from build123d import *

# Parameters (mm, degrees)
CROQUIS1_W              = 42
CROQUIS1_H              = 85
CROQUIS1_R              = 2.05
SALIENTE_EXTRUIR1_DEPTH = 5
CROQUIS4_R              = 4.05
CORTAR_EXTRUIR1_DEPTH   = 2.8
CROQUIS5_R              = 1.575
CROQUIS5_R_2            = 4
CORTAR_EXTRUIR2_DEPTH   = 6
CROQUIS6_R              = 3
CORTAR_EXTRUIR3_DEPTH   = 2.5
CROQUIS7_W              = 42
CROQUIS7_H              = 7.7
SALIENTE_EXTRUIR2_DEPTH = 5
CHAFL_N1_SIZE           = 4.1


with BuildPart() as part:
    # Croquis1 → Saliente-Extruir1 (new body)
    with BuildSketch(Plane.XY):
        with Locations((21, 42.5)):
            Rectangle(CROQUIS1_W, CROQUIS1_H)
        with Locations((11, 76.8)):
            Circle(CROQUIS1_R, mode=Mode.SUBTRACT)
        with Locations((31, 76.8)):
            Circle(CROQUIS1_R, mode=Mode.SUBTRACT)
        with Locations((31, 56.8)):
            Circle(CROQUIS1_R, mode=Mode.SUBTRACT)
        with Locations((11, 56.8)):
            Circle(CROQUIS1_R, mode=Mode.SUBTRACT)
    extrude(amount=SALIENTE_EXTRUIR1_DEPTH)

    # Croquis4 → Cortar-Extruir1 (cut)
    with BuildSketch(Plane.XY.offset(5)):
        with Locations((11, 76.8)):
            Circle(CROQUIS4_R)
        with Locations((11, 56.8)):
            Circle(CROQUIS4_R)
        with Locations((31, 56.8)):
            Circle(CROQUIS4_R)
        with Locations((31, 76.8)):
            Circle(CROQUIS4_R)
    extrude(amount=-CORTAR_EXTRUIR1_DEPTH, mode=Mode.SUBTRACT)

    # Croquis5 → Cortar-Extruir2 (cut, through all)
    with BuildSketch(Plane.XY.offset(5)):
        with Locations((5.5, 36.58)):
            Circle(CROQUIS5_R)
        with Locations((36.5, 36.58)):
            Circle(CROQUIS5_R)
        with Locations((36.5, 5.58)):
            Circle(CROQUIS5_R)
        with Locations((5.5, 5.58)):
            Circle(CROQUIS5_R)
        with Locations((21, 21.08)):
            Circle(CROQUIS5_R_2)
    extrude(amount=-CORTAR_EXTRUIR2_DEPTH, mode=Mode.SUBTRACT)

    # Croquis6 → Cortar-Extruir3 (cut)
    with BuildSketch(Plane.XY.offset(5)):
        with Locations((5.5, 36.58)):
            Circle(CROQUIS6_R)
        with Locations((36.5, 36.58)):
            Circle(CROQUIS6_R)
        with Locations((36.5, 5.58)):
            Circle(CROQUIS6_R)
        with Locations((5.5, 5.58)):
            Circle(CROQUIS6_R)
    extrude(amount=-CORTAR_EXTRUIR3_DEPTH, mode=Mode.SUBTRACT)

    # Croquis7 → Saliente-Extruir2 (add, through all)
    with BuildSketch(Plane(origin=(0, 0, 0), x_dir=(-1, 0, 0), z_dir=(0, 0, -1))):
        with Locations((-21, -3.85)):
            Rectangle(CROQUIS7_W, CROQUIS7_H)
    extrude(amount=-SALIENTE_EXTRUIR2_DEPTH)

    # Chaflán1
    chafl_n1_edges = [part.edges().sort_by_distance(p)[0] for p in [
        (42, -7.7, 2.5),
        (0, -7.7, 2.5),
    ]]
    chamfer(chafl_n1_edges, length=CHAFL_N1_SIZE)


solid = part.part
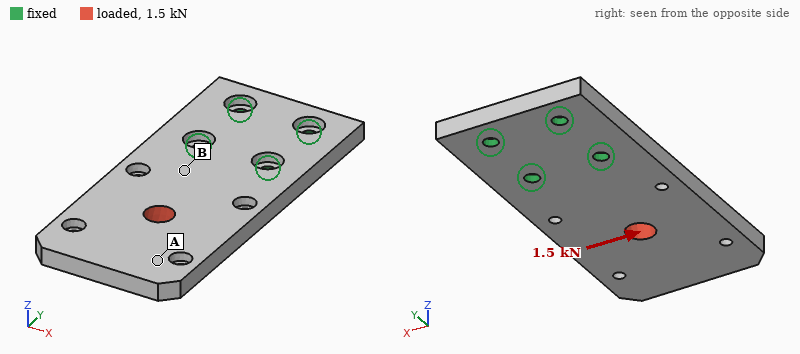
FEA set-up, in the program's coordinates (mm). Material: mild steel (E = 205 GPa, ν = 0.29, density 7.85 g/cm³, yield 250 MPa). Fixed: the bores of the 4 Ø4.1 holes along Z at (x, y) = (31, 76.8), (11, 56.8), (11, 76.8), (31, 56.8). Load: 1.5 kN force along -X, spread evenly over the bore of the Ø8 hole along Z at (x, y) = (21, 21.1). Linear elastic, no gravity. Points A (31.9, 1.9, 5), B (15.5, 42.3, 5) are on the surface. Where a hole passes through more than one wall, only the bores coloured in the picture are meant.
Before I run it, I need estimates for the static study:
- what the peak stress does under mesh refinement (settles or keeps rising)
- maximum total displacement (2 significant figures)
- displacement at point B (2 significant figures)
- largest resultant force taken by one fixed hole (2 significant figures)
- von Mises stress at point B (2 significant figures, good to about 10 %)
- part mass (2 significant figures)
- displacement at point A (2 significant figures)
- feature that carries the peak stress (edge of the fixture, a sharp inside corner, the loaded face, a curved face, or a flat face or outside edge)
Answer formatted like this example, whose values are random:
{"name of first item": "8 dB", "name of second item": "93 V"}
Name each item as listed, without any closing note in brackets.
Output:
{"what the peak stress does under mesh refinement": "keeps rising", "maximum total displacement": "20 µm", "displacement at point B": "4.1 µm", "largest resultant force taken by one fixed hole": "1.7 kN", "von Mises stress at point B": "18 MPa", "part mass": "140 g", "displacement at point A": "17 µm", "feature that carries the peak stress": "edge of the fixture"}
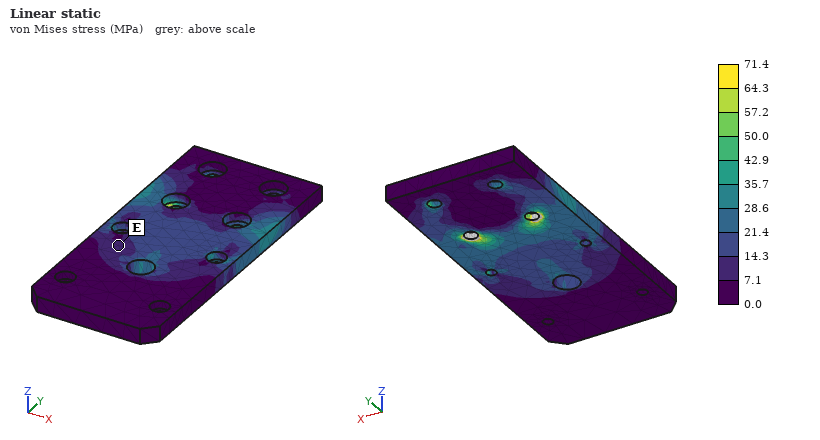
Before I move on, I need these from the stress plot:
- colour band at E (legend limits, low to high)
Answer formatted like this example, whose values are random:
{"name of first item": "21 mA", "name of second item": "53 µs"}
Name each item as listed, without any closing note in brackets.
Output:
{"colour band at E": "7.1 to 14.3 MPa"}
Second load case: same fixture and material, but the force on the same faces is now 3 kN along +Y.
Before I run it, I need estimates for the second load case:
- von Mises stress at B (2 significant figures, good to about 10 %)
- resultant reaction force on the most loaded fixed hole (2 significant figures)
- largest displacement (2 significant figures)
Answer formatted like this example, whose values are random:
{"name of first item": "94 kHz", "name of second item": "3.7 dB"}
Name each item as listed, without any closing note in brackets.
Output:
{"von Mises stress at B": "19 MPa", "resultant reaction force on the most loaded fixed hole": "1.1 kN", "largest displacement": "20 µm"}
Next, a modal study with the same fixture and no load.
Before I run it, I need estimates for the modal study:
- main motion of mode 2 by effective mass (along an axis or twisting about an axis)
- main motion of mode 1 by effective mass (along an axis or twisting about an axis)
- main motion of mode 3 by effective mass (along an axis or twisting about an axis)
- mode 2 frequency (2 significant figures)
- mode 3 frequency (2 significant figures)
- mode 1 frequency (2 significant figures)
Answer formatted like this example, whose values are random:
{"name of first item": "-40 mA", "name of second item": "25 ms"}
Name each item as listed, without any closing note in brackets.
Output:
{"main motion of mode 2 by effective mass": "twisting about Y", "main motion of mode 1 by effective mass": "along Z", "main motion of mode 3 by effective mass": "along X", "mode 2 frequency": "3100 Hz", "mode 3 frequency": "5300 Hz", "mode 1 frequency": "890 Hz"}
